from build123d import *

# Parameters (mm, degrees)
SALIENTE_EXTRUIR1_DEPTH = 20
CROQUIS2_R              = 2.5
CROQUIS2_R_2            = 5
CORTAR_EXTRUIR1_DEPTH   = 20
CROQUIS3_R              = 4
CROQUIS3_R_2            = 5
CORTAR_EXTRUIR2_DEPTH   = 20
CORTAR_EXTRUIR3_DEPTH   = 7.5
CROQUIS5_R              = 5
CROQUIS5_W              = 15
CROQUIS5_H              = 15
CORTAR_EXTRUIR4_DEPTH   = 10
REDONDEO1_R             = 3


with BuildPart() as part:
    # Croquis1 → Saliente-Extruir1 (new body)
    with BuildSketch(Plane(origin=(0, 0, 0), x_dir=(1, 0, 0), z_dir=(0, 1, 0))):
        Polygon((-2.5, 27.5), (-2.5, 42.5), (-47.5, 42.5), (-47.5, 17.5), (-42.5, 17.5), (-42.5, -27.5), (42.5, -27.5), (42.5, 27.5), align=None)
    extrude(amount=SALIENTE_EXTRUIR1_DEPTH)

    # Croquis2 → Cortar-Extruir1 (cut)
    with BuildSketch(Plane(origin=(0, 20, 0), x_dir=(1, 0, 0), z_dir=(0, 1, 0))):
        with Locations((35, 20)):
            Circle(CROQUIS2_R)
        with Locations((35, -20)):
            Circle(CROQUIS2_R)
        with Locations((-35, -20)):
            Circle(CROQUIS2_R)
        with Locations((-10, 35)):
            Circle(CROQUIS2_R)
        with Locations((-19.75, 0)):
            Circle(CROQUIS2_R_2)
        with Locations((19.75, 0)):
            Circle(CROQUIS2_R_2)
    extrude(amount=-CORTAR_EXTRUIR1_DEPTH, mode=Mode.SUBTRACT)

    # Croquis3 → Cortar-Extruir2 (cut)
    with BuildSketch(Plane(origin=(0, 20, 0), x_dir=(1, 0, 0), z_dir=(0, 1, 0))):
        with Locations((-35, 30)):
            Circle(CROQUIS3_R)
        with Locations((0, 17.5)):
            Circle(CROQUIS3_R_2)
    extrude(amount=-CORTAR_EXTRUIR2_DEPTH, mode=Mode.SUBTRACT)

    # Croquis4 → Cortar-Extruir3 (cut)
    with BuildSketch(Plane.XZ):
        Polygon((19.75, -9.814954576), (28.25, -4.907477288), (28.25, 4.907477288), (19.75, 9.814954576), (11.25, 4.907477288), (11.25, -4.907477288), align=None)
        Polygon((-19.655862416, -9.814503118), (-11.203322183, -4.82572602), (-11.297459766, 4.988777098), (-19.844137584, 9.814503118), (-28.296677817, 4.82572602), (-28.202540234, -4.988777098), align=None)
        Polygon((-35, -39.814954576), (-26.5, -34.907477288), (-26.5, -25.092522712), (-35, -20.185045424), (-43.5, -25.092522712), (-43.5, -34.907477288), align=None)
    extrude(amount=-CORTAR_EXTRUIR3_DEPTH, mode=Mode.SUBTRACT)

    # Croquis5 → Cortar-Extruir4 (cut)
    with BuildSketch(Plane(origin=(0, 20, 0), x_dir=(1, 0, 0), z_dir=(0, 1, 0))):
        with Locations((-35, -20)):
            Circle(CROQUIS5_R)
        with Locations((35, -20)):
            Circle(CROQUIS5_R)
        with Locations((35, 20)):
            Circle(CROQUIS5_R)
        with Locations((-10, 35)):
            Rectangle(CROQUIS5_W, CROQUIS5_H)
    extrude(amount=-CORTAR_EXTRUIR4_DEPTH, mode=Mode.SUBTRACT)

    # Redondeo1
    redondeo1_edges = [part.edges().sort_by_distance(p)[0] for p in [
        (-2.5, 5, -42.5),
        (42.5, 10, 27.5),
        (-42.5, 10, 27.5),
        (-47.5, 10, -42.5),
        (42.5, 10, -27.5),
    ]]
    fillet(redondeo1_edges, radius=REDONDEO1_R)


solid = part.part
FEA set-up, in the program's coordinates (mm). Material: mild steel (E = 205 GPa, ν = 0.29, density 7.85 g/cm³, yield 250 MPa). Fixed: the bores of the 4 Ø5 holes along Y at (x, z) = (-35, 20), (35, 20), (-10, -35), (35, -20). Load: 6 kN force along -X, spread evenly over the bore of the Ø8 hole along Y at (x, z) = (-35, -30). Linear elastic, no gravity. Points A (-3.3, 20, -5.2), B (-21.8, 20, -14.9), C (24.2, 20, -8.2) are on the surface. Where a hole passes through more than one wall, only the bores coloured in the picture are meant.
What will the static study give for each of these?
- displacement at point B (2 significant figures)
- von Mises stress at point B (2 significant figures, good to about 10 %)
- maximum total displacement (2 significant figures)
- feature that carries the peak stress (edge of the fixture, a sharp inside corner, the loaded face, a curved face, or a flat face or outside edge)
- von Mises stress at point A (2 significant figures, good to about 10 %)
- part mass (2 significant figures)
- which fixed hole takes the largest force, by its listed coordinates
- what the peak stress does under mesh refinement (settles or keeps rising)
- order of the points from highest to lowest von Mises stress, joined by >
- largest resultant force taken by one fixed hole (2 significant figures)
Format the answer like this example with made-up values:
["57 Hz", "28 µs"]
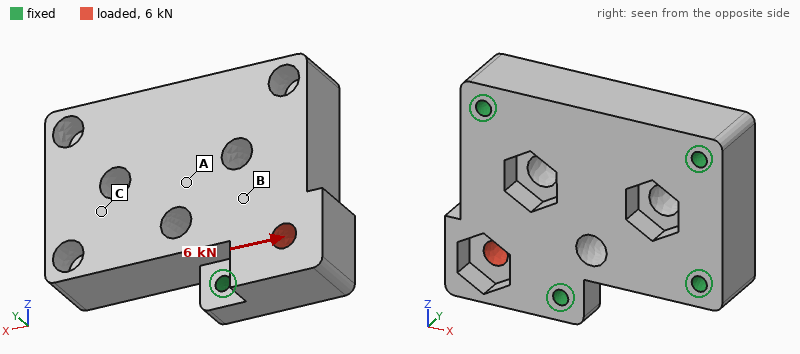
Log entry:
["3.2 µm", "18 MPa", "11 µm", "edge of the fixture", "9.0 MPa", "730 g", "(-10, -35)", "keeps rising", "B > A > C", "3.5 kN"]
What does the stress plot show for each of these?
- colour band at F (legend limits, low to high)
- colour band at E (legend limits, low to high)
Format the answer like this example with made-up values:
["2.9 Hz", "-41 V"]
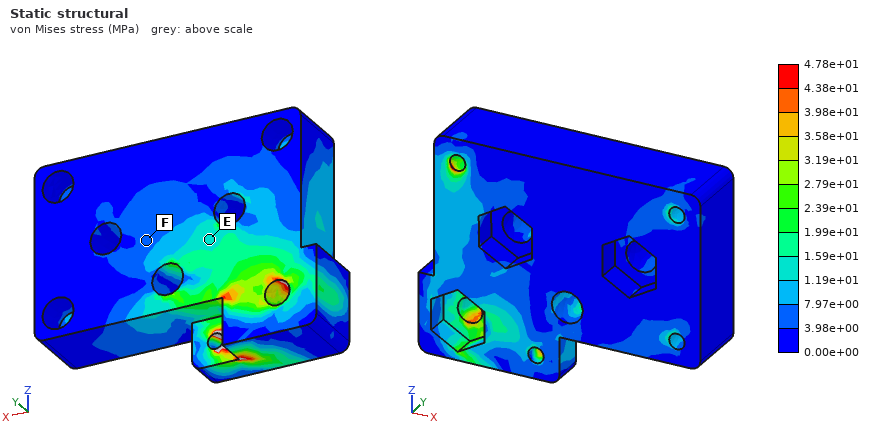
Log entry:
["3.98e+00 to 7.97e+00 MPa", "1.19e+01 to 1.59e+01 MPa"]
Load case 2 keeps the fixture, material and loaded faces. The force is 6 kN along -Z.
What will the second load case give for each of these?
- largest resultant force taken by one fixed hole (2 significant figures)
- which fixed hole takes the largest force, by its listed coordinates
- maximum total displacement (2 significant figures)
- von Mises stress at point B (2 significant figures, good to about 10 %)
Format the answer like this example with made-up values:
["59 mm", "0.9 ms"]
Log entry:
["3.4 kN", "(-35, 20)", "5.7 µm", "9.3 MPa"]
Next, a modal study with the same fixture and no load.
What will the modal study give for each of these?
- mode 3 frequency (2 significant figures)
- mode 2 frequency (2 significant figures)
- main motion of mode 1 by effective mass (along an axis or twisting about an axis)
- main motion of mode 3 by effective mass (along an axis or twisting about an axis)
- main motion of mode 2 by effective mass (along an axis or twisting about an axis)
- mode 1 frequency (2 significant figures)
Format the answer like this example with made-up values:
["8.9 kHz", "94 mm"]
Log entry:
["15 kHz", "11 kHz", "along Y", "along Z", "along Y", "8000 Hz"]
